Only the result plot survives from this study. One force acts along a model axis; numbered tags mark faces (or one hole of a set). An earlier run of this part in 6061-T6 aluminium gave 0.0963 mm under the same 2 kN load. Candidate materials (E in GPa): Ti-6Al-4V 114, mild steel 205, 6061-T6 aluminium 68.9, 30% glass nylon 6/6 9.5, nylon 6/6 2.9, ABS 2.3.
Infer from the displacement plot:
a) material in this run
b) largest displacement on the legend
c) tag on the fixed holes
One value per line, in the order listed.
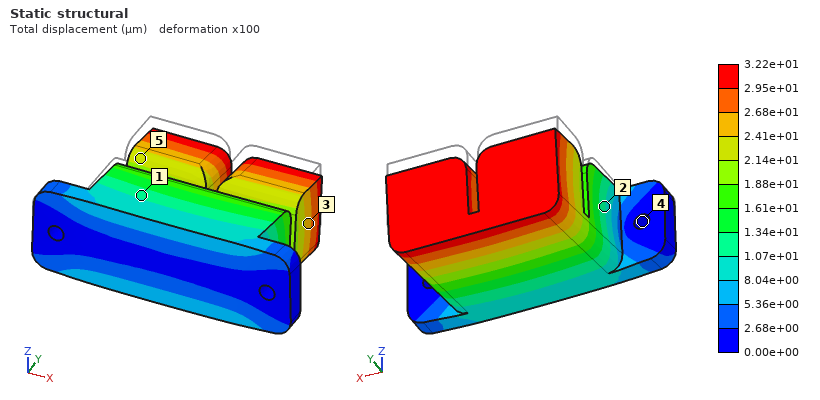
mild steel
3.22e+01 µm
4
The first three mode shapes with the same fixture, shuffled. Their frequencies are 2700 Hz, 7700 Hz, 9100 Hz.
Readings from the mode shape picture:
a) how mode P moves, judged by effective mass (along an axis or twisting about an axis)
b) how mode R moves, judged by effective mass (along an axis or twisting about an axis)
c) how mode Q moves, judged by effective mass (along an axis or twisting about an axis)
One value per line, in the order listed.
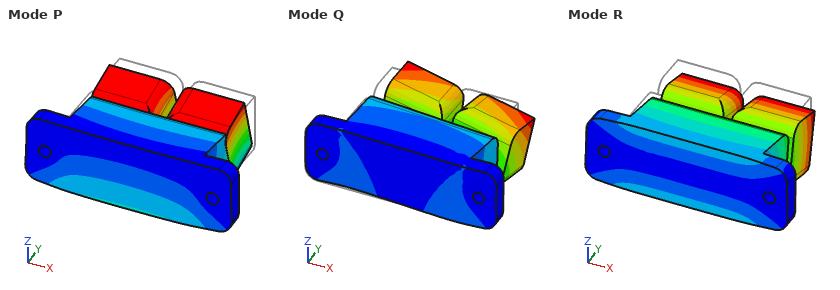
along Y
along Z
along X
